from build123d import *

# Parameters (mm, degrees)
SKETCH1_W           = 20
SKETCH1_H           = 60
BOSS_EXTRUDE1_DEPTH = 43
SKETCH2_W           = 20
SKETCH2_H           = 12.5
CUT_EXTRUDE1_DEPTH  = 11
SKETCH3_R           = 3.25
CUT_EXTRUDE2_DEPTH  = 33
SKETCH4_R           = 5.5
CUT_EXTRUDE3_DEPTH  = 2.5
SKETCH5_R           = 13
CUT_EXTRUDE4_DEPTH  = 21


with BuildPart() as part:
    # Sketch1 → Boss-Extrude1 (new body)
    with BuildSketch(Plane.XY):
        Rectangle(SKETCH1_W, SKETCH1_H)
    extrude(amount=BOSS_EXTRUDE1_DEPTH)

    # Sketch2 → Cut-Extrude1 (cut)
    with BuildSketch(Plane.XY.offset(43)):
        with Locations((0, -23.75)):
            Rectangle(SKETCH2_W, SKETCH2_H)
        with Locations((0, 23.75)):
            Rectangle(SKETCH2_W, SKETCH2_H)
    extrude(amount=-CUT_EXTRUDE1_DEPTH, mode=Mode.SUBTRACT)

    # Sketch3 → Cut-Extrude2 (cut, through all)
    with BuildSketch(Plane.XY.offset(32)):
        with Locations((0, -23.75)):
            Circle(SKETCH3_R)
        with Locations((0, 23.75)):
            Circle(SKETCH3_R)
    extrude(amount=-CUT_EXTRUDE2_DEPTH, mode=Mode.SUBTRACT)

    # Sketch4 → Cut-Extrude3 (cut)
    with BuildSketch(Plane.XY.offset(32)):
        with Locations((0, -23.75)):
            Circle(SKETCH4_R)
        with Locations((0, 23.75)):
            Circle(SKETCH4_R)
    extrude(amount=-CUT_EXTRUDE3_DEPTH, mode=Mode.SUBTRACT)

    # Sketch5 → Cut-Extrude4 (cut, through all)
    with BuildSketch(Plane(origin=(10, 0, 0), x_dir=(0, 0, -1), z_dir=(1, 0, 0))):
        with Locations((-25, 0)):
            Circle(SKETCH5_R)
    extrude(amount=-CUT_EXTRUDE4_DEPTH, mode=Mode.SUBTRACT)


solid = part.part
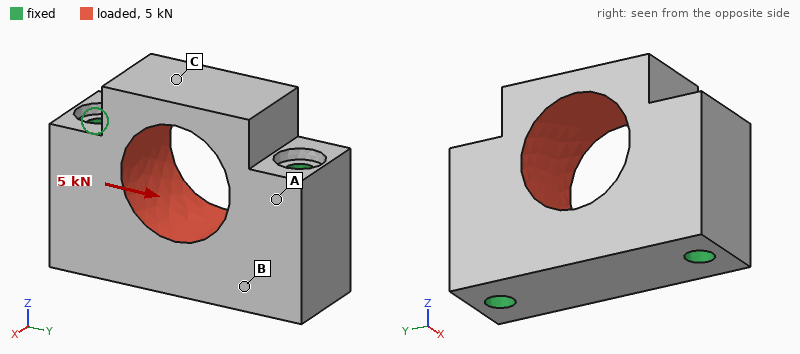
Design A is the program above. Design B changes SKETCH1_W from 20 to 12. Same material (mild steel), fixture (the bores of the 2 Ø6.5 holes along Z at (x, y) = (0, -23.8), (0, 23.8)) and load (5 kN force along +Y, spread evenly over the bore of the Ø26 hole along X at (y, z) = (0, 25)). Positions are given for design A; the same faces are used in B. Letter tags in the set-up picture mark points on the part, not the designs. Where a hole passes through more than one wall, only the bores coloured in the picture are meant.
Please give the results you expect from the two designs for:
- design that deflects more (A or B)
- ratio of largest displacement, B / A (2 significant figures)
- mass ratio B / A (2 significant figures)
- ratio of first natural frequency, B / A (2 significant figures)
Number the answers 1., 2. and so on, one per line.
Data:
1. B
2. 1.7
3. 0.57
4. 0.82
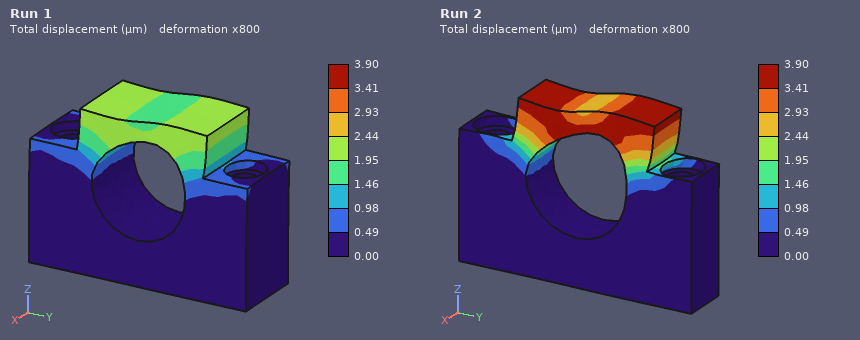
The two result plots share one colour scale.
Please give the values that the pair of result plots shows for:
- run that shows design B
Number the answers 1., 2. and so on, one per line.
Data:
1. Run 2
